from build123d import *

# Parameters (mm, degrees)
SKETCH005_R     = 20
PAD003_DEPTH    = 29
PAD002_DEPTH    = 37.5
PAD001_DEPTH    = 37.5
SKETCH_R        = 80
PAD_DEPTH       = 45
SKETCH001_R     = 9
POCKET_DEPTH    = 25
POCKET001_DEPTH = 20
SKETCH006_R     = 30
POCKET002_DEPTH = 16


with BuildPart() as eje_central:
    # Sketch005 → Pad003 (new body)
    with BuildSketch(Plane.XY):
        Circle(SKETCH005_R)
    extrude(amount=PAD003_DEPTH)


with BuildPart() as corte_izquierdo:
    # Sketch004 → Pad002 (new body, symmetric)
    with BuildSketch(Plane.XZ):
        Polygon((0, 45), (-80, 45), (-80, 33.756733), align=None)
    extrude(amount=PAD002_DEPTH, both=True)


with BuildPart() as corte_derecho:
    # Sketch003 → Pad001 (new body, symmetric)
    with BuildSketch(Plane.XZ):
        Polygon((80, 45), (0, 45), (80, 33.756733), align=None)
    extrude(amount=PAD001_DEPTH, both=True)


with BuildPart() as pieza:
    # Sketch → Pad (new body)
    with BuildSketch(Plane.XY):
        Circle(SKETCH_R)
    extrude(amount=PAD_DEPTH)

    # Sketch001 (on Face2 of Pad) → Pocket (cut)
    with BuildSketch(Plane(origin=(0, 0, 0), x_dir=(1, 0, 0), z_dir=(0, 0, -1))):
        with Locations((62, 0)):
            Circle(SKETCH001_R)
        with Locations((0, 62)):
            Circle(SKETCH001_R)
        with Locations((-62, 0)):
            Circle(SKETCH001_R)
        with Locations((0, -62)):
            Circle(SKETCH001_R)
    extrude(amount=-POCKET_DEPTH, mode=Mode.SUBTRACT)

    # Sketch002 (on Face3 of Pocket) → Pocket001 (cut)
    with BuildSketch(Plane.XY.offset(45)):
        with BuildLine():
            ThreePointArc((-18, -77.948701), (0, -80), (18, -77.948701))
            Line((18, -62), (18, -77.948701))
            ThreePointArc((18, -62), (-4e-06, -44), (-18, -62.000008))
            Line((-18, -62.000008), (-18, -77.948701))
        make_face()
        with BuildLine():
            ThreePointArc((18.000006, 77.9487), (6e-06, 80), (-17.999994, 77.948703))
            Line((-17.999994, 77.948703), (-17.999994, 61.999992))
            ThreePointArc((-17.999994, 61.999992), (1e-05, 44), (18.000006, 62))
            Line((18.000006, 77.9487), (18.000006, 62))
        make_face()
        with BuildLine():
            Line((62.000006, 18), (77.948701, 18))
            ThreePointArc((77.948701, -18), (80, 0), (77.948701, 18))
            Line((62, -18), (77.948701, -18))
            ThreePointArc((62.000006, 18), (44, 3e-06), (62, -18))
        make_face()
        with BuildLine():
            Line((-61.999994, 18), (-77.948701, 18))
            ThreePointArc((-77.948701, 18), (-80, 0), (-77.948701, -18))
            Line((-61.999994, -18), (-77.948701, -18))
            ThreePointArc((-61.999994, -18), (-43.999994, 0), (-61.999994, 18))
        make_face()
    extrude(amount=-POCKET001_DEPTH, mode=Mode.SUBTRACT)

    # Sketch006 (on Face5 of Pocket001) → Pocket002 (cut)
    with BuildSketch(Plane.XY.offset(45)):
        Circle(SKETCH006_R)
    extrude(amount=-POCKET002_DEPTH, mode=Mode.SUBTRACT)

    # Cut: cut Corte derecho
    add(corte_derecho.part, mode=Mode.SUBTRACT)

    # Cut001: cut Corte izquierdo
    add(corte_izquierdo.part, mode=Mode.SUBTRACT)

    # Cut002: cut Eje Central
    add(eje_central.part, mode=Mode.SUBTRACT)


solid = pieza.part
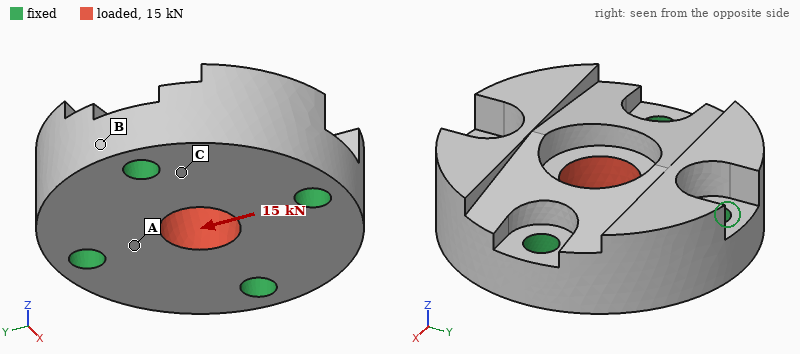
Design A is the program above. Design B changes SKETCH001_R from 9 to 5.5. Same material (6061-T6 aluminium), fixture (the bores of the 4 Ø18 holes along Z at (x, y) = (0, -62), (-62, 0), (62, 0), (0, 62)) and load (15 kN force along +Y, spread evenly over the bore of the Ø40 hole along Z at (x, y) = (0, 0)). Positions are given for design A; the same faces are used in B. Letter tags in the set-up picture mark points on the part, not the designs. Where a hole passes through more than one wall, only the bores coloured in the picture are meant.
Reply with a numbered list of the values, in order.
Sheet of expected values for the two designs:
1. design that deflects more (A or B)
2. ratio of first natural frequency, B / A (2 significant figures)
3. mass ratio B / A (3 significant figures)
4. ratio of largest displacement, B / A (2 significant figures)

1. B
2. 0.85
3. 1.02
4. 1.1
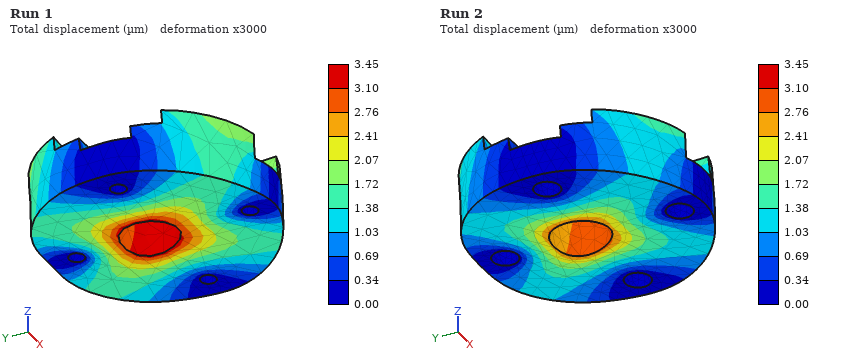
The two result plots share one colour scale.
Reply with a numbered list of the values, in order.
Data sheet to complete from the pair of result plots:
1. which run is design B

1. Run 1
